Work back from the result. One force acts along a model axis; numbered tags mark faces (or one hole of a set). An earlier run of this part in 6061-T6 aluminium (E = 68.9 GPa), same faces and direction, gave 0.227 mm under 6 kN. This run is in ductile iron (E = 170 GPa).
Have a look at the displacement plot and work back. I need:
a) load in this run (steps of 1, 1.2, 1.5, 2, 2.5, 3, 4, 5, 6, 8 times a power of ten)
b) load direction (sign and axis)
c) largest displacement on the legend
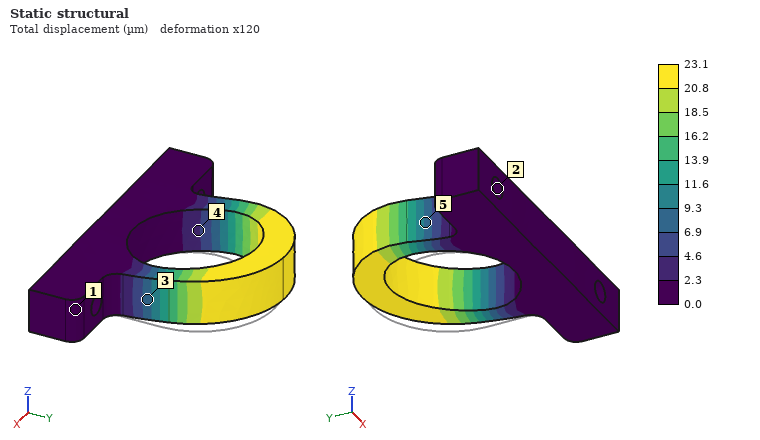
1.5 kN
-X
23.1 µm
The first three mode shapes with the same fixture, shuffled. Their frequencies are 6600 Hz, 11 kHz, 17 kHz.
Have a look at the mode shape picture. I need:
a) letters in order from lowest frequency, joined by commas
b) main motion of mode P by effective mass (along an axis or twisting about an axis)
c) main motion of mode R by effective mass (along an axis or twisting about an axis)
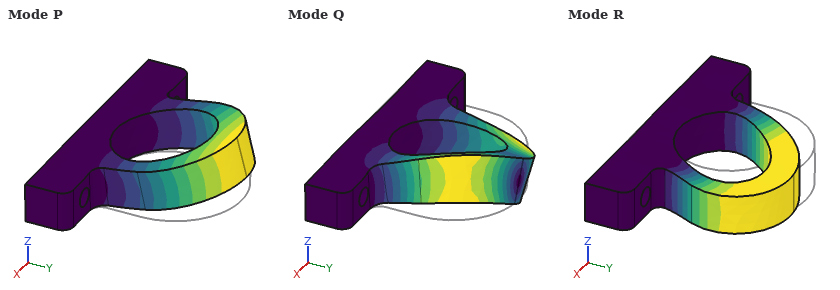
P, R, Q
along Z
along X
